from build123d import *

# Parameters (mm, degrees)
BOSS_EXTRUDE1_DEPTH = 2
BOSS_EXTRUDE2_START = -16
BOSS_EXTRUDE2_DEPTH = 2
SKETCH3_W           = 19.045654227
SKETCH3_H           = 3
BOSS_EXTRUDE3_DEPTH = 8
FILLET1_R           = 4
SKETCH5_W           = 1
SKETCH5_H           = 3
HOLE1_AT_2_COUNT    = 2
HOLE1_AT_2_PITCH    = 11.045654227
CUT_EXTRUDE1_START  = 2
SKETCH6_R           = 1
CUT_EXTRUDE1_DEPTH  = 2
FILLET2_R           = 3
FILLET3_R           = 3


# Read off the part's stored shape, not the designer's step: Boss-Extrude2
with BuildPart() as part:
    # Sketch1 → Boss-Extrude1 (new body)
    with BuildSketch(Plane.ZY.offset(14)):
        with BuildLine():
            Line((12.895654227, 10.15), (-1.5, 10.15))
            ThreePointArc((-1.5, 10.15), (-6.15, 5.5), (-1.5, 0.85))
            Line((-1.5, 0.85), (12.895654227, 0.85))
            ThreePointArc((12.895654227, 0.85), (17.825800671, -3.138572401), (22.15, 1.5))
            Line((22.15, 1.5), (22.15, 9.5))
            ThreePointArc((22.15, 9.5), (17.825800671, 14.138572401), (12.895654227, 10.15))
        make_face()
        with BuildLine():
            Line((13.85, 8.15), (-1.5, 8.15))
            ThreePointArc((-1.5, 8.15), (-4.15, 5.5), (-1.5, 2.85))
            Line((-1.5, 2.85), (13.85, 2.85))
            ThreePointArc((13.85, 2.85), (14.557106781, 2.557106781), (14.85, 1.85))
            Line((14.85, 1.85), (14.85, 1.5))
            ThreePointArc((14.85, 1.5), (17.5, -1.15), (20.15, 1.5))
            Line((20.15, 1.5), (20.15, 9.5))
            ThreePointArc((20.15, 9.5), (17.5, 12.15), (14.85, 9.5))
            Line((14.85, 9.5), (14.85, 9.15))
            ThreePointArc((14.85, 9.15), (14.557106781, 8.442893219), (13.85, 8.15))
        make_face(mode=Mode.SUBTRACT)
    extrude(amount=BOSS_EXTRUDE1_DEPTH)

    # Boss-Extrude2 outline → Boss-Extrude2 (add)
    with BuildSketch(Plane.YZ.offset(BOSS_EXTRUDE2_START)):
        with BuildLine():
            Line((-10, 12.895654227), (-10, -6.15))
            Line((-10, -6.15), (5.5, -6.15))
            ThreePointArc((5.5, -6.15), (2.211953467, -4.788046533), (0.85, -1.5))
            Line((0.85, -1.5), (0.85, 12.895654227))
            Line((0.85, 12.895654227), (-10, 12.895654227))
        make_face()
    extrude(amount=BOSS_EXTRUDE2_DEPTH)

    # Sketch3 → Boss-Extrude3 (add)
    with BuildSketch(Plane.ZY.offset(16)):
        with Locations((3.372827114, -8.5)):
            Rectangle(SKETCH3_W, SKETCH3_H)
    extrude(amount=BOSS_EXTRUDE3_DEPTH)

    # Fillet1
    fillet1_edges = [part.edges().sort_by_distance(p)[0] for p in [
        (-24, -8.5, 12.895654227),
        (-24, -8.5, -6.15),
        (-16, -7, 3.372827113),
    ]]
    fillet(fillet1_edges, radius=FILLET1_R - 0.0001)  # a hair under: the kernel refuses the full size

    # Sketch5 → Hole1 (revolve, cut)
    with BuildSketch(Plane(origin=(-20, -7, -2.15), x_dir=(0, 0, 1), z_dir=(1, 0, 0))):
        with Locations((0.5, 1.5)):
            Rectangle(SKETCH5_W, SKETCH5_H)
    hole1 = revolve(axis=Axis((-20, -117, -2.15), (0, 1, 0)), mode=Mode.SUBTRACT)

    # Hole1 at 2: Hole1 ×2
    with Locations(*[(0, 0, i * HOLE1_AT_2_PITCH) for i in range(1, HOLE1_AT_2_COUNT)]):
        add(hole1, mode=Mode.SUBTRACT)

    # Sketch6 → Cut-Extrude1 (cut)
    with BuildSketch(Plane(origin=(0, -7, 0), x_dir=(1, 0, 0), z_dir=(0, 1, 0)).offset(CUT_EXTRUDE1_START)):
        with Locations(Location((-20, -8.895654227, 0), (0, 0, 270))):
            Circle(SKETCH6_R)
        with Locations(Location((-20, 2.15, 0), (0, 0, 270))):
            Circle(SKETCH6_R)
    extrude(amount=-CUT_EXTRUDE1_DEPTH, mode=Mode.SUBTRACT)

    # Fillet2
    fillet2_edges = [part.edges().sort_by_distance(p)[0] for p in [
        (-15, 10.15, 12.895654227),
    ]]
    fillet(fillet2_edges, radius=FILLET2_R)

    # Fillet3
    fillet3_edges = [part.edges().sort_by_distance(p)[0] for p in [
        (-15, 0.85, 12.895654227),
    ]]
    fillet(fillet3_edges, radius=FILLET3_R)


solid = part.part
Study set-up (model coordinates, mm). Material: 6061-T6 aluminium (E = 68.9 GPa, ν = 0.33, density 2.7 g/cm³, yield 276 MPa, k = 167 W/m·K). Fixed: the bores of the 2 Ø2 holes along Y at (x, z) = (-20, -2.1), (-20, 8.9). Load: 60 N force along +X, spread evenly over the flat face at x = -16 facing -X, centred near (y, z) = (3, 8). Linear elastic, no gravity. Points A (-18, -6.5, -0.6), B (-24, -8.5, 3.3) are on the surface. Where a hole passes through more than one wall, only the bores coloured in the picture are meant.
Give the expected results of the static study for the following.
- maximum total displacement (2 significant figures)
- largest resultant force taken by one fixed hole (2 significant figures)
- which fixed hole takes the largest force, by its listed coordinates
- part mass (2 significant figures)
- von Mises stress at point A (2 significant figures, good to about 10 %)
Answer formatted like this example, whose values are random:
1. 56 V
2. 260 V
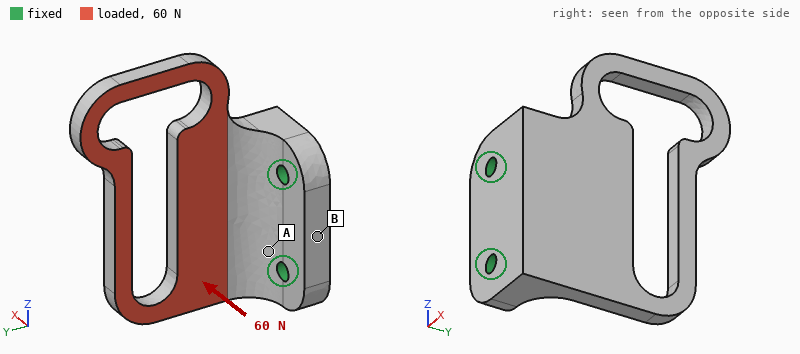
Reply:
1. 0.28 mm
2. 50 N
3. (-20, 8.9)
4. 3.3 g
5. 19 MPa
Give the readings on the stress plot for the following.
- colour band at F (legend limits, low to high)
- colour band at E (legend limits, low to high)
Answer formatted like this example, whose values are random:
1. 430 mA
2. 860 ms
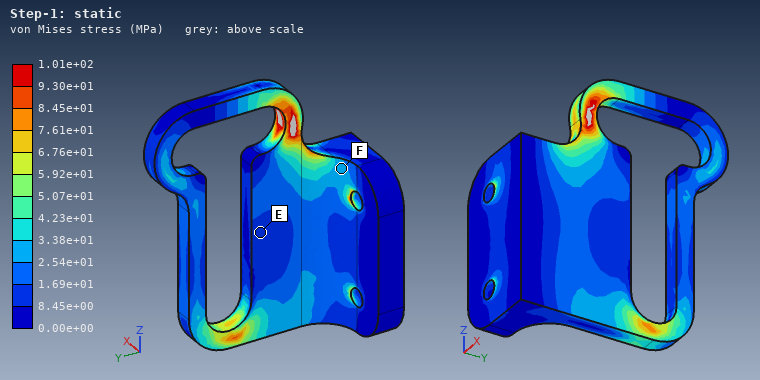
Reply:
1. 2.54e+01 to 3.38e+01 MPa
2. 8.45e+00 to 1.69e+01 MPa
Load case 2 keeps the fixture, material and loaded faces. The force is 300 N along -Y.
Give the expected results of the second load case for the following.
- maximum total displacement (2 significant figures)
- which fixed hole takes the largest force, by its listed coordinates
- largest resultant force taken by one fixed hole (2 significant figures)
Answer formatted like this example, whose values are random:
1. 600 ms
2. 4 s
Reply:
1. 0.16 mm
2. (-20, 8.9)
3. 240 N
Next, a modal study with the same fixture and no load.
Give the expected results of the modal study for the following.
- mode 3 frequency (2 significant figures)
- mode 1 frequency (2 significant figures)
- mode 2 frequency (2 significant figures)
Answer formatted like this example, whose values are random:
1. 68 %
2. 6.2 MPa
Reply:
1. 7600 Hz
2. 2700 Hz
3. 7100 Hz
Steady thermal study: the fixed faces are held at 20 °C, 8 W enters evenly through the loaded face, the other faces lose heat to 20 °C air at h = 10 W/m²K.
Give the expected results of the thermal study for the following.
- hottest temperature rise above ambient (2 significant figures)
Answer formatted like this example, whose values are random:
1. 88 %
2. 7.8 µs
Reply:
1. 47 K
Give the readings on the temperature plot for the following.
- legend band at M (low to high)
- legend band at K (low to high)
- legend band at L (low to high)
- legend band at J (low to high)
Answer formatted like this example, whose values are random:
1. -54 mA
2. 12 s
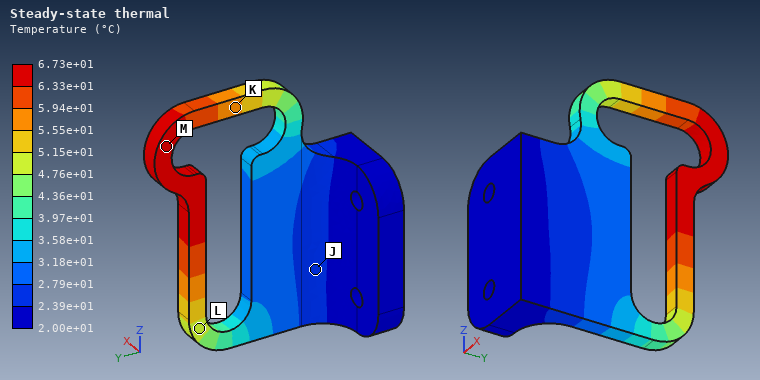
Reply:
1. 6.33e+01 to 6.73e+01 °C
2. 5.55e+01 to 5.94e+01 °C
3. 4.76e+01 to 5.15e+01 °C
4. 2.39e+01 to 2.79e+01 °C
